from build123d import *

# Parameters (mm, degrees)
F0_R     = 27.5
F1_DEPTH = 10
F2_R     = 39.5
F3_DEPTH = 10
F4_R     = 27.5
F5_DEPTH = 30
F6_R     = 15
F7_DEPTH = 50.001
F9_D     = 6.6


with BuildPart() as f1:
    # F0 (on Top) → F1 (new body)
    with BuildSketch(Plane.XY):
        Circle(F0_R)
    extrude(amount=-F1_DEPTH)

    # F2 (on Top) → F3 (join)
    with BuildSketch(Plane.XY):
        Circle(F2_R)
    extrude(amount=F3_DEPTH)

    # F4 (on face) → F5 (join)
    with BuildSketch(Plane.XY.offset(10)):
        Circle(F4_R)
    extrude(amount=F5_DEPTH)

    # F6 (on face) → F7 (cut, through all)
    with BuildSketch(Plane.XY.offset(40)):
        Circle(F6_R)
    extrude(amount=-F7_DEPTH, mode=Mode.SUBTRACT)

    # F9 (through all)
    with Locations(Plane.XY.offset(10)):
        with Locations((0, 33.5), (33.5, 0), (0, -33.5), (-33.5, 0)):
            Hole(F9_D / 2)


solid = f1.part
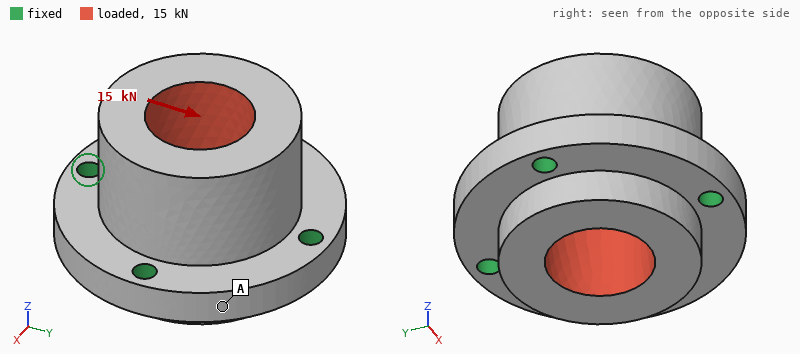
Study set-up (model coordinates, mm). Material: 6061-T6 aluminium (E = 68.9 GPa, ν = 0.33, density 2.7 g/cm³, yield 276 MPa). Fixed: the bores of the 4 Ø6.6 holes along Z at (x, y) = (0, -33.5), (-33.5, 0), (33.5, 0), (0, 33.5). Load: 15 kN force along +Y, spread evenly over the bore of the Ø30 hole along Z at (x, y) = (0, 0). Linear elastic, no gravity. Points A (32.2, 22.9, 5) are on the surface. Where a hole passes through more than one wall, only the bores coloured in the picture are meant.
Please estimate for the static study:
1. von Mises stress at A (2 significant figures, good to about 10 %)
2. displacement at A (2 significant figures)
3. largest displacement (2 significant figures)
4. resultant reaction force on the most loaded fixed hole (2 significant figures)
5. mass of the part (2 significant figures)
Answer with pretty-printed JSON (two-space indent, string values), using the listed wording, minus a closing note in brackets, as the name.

{
  "von Mises stress at A": "7.3 MPa",
  "displacement at A": "4.7 µm",
  "largest displacement": "18 µm",
  "resultant reaction force on the most loaded fixed hole": "4.9 kN",
  "mass of the part": "290 g"
}
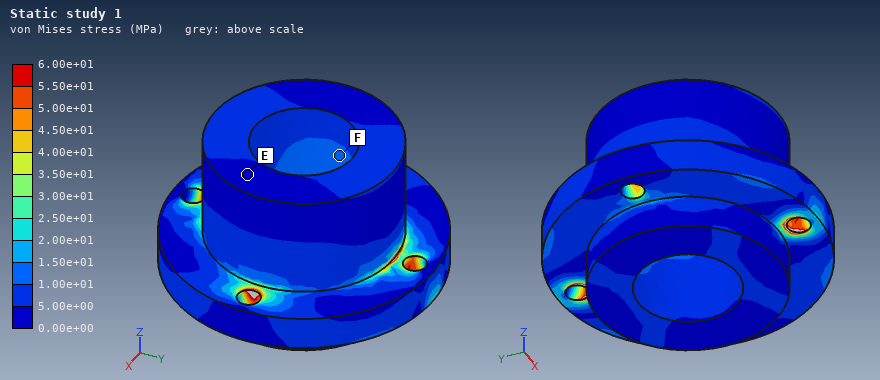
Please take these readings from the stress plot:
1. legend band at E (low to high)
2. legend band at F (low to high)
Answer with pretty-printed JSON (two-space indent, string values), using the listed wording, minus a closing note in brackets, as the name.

{
  "legend band at E": "0.00e+00 to 5.00e+00 MPa",
  "legend band at F": "1.00e+01 to 1.50e+01 MPa"
}
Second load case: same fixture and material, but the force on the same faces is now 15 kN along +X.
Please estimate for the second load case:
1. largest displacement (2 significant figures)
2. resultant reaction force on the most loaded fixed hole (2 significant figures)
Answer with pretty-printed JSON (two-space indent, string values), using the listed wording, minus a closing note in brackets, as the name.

{
  "largest displacement": "18 µm",
  "resultant reaction force on the most loaded fixed hole": "4.9 kN"
}
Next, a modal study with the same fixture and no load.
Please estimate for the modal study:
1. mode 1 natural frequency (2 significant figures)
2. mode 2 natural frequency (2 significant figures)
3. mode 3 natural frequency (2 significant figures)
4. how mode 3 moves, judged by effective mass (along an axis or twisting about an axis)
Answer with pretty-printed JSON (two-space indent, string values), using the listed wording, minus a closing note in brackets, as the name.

{
  "mode 1 natural frequency": "11 kHz",
  "mode 2 natural frequency": "11 kHz",
  "mode 3 natural frequency": "13 kHz",
  "how mode 3 moves, judged by effective mass": "along Z"
}
